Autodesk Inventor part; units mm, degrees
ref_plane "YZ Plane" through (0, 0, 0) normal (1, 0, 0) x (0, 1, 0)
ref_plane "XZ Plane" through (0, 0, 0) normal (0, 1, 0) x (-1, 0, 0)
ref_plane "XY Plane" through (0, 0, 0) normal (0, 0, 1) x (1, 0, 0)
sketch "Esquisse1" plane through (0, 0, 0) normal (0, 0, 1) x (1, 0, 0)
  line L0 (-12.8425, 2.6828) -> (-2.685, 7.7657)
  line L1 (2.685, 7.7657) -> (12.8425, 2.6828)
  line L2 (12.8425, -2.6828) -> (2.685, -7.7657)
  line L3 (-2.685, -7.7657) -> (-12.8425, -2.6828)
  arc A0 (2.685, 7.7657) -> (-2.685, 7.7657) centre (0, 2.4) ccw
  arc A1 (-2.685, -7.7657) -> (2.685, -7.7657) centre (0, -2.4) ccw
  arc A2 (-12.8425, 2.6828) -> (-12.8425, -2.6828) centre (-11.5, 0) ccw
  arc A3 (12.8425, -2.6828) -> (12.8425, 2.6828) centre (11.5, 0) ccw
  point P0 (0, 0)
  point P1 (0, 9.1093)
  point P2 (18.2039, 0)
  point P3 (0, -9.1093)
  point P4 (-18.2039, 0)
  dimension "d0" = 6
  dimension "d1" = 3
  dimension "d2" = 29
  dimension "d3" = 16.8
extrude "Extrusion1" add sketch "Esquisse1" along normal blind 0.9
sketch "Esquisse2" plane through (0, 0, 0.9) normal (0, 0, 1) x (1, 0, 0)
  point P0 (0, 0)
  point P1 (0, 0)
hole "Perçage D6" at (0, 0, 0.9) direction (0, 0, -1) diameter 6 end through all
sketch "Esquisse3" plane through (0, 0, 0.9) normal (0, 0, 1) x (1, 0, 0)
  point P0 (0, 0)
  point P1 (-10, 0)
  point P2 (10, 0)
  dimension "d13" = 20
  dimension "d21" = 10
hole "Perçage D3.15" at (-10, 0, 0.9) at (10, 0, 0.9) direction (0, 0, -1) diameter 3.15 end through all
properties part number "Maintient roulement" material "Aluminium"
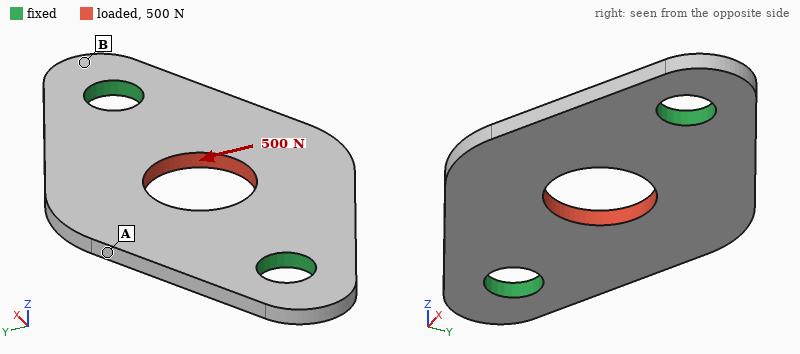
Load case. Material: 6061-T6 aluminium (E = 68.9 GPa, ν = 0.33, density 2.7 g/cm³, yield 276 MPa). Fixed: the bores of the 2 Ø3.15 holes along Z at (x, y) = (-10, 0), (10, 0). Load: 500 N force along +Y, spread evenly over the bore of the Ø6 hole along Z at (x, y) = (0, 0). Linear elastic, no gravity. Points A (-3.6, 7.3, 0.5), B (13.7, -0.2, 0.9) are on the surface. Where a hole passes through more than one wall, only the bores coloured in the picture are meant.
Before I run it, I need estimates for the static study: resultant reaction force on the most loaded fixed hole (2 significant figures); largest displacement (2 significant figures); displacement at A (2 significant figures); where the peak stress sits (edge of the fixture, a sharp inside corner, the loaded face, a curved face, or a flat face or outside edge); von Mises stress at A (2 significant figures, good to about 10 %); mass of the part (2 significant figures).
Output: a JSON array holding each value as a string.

["250 N", "10 µm", "7.7 µm", "edge of the fixture", "50 MPa", "0.65 g"]
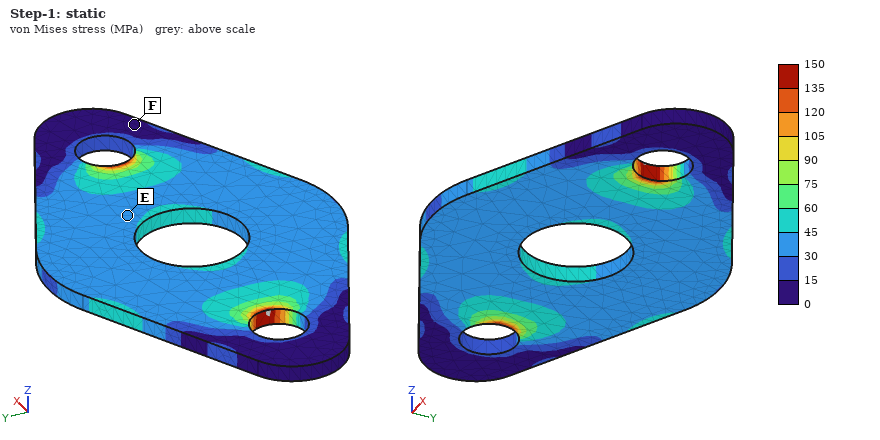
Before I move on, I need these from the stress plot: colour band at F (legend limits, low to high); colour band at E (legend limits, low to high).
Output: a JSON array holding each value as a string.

["0 to 15 MPa", "30 to 45 MPa"]
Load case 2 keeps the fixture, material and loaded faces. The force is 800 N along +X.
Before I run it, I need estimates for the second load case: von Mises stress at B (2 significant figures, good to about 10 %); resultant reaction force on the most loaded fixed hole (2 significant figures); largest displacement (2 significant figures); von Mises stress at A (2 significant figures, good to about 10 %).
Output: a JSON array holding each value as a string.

["11 MPa", "400 N", "7.4 µm", "10 MPa"]
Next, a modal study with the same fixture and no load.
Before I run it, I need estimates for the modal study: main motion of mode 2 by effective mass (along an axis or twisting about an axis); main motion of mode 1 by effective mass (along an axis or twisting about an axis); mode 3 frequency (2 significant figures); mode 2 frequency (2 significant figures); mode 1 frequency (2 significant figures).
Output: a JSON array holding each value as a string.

["along Z", "twisting about X", "27 kHz", "10 kHz", "9600 Hz"]
